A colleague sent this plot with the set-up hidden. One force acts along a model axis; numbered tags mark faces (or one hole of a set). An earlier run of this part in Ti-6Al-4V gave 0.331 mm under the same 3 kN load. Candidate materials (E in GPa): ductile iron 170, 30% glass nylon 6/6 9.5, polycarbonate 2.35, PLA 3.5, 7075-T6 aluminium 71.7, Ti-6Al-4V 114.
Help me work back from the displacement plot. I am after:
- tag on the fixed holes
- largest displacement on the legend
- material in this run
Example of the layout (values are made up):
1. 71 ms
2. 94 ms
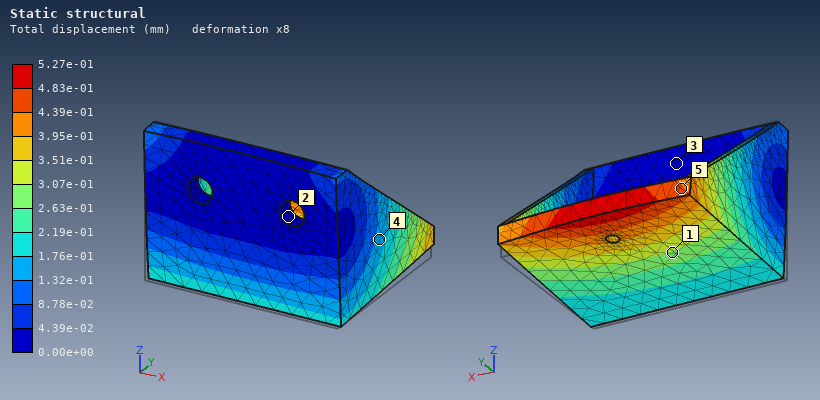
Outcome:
1. 2
2. 5.27e-01 mm
3. 7075-T6 aluminium
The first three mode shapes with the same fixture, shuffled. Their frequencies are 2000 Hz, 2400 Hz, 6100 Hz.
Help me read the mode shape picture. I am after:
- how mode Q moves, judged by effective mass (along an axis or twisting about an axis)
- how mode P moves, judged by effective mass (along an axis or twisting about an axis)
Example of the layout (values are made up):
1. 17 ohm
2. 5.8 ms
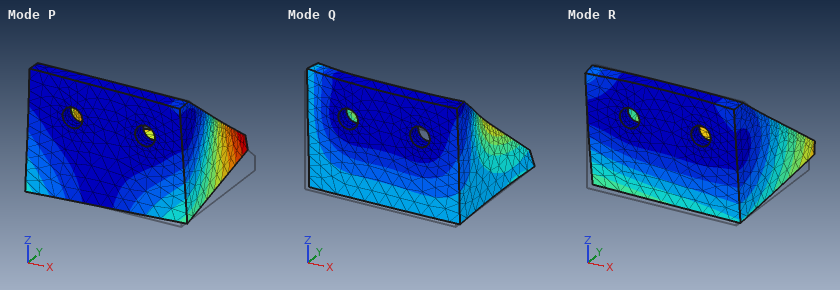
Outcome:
1. along Y
2. along X
